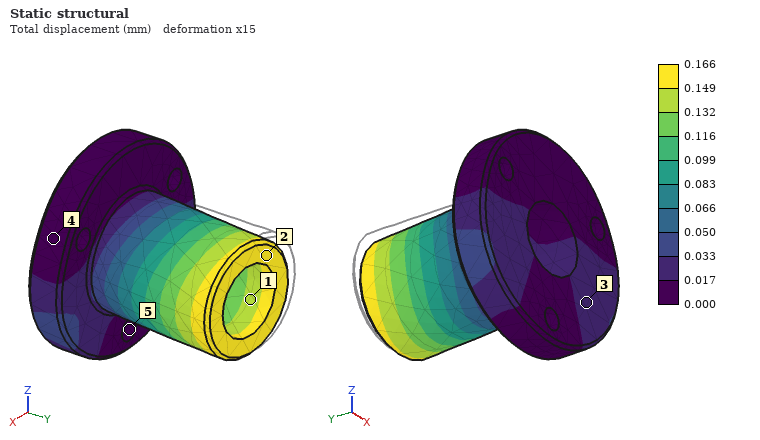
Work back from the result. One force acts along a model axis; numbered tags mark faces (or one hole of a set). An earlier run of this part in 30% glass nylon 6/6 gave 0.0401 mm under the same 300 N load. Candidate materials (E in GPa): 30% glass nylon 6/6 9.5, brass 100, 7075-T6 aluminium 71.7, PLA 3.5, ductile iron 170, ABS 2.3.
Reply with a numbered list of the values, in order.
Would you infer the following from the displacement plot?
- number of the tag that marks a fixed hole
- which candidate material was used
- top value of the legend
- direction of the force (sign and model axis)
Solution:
1. 5
2. ABS
3. 0.166 mm
4. +X
